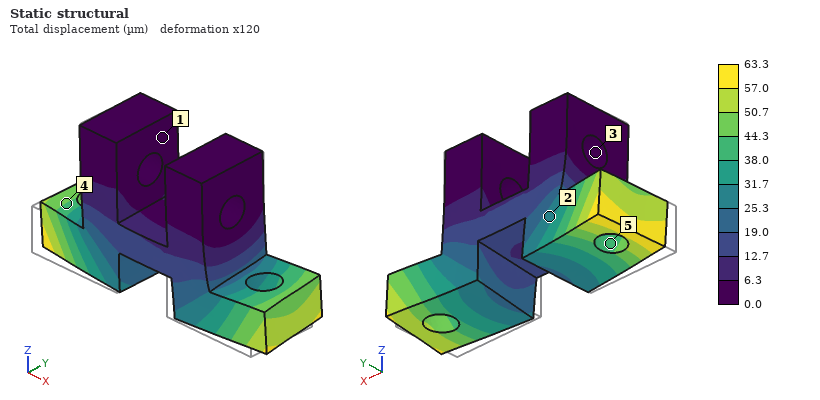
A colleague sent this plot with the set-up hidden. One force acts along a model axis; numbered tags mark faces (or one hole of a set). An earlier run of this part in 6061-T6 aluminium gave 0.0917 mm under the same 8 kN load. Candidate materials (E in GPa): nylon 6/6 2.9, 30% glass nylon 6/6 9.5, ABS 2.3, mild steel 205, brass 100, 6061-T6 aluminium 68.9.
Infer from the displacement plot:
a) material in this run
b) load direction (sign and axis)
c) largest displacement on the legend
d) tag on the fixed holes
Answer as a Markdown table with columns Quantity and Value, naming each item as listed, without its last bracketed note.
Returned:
| Quantity | Value |
|---|---|
| material in this run | brass |
| load direction | +Y |
| largest displacement on the legend | 63.3 µm |
| tag on the fixed holes | 3 |
